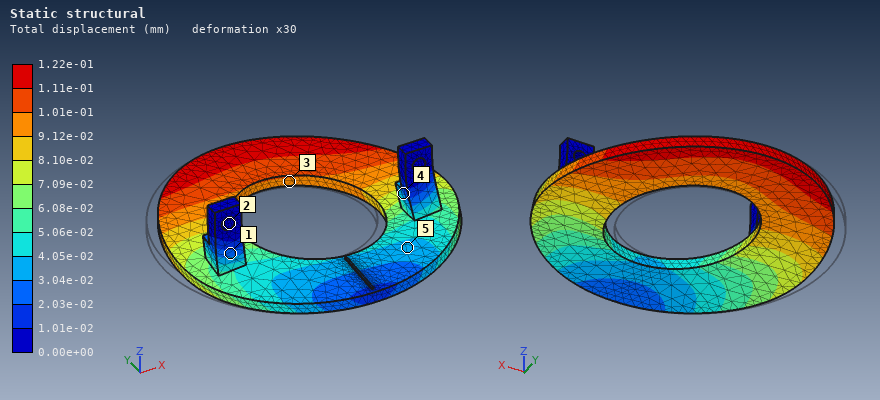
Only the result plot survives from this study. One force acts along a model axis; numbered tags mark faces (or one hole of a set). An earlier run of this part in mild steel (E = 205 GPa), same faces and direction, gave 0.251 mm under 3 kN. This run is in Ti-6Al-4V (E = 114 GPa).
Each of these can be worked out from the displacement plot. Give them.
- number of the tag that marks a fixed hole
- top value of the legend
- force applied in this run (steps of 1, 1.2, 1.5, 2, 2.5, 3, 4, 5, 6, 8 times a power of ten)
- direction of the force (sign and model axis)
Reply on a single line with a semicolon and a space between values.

2; 1.22e-01 mm; 800 N; +X
